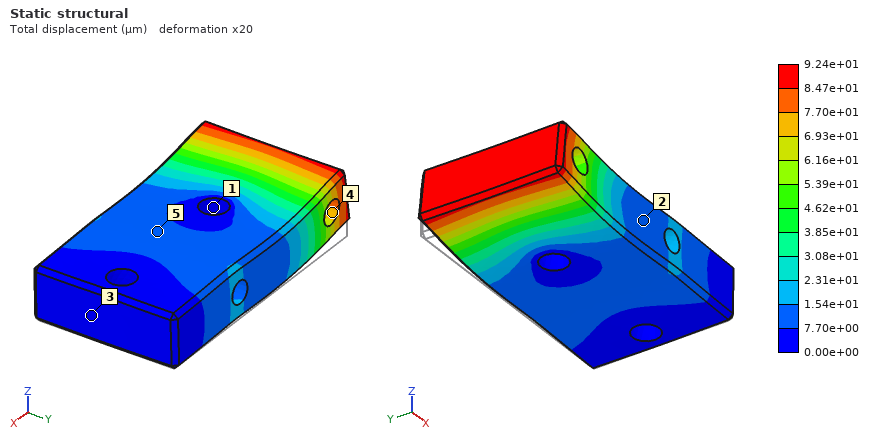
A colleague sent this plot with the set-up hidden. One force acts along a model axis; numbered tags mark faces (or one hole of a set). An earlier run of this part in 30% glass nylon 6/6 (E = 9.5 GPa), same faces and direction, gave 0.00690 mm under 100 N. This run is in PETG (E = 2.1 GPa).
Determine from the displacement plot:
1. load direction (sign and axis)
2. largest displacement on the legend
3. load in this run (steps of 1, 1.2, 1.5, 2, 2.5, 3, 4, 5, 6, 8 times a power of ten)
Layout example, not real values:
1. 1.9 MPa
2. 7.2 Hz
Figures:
1. +Z
2. 9.24e+01 µm
3. 300 N
